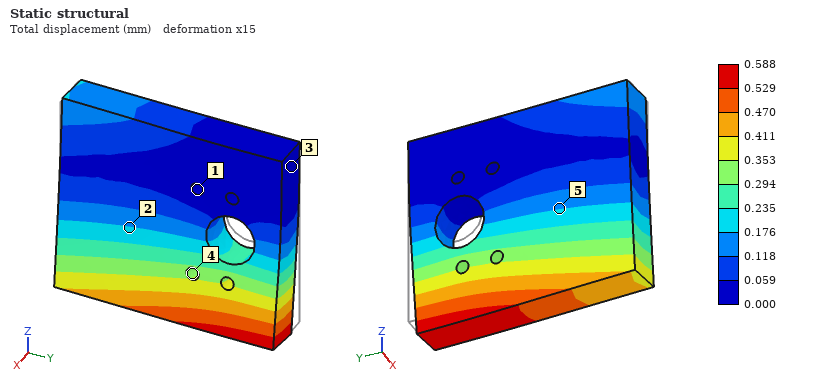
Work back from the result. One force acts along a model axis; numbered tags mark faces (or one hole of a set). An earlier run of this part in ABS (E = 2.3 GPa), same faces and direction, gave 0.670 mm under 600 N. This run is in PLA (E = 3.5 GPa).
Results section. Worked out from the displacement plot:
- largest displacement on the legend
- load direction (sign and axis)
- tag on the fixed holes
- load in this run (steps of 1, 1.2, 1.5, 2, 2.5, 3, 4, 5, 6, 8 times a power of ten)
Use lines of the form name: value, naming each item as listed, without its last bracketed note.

largest displacement on the legend: 0.588 mm
load direction: +X
tag on the fixed holes: 1
load in this run: 800 N
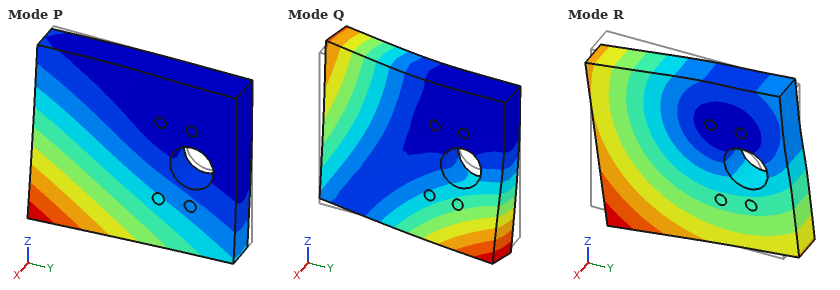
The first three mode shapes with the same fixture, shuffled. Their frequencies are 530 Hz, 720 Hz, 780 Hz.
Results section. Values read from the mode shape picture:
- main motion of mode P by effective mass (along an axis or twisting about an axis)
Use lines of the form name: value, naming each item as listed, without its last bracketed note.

main motion of mode P by effective mass: along X
